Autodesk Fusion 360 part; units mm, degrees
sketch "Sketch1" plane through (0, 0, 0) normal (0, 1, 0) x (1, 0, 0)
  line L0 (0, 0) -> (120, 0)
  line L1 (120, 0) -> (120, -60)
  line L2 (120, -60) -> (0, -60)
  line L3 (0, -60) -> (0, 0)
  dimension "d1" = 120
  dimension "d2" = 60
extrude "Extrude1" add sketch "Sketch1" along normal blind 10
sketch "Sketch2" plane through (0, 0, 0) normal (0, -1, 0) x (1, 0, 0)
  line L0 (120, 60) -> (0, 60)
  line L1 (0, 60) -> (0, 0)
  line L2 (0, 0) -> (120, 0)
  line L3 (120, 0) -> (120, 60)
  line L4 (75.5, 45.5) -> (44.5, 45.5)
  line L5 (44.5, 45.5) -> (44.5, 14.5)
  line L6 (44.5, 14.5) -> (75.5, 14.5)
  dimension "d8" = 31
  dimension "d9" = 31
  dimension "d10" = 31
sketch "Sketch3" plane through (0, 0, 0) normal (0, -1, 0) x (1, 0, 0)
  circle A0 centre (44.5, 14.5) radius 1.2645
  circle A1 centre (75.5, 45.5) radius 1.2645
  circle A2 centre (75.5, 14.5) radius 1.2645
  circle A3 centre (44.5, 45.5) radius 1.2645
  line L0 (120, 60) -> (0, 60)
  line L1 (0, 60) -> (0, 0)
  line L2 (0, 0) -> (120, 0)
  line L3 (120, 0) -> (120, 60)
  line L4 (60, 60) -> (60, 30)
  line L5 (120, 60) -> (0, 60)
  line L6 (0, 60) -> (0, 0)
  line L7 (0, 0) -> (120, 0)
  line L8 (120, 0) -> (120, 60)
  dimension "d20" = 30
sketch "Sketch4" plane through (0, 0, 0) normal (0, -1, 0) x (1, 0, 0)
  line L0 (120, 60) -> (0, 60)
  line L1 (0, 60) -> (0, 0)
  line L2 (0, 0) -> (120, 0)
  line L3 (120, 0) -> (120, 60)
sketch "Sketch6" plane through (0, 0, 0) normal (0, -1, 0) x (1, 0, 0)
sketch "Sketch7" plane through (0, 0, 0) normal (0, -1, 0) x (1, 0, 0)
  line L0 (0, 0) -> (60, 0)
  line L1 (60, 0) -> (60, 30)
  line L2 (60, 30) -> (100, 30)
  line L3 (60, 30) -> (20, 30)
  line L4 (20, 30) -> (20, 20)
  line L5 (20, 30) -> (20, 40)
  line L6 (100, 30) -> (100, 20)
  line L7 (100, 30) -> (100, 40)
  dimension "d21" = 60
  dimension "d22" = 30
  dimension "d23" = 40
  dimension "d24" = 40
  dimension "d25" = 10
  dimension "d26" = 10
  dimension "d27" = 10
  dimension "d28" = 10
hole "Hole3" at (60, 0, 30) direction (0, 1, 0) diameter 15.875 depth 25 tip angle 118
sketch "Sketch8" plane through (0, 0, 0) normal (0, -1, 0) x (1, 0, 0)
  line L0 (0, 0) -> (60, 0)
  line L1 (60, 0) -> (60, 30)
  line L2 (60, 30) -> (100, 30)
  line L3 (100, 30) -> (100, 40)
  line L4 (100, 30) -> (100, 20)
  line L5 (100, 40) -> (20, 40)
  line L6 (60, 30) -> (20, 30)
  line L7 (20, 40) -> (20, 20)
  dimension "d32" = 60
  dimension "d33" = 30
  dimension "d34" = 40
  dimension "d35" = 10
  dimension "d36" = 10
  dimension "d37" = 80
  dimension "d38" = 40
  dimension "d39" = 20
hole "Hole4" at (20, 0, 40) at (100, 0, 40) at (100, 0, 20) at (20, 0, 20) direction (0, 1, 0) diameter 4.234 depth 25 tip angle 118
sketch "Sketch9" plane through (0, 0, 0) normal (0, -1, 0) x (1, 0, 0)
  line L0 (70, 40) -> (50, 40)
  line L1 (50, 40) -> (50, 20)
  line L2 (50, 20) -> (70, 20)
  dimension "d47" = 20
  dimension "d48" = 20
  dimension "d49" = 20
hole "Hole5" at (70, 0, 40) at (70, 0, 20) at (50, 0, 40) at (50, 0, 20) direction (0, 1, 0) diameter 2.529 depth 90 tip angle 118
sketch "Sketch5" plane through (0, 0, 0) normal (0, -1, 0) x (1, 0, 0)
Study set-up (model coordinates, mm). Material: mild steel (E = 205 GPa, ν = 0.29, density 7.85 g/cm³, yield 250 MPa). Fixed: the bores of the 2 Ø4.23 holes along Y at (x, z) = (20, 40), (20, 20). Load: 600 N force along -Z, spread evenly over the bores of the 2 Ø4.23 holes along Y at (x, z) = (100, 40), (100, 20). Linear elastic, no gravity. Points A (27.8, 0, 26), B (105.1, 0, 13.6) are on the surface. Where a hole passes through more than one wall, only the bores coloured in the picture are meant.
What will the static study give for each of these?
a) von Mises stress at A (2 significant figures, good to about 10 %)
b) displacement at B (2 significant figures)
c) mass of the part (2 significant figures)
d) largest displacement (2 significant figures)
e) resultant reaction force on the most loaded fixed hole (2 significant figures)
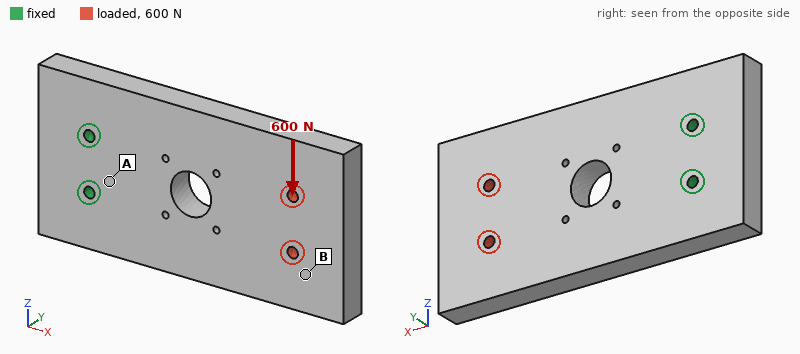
8.5 MPa
9.5 µm
540 g
11 µm
2.1 kN
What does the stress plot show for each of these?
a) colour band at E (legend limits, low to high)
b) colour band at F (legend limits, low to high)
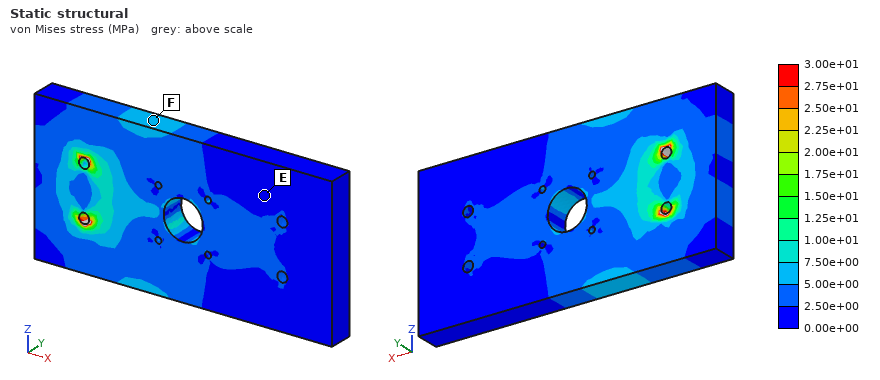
0.00e+00 to 2.50e+00 MPa
5.00e+00 to 7.50e+00 MPa
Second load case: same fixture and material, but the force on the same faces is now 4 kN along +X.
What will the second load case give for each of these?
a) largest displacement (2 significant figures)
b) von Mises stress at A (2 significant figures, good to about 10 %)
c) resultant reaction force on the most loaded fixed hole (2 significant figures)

4.1 µm
6.2 MPa
2.0 kN
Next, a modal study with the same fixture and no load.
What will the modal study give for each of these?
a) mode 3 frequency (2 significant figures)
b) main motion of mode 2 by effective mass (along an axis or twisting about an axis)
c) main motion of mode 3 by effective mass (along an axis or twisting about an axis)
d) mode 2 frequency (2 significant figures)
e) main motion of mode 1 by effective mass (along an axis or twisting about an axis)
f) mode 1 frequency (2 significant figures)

2600 Hz
twisting about X
along Z
2500 Hz
along Y
760 Hz
